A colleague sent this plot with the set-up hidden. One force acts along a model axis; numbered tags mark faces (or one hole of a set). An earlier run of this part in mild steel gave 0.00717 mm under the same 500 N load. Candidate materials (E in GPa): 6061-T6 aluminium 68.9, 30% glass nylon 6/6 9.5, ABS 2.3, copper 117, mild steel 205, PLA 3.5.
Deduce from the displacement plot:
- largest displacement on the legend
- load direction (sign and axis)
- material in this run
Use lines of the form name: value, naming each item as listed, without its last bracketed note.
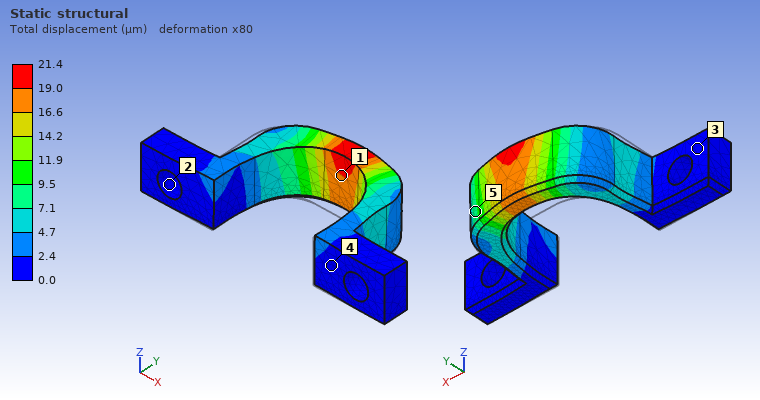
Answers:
largest displacement on the legend: 21.4 µm
load direction: +Y
material in this run: 6061-T6 aluminium
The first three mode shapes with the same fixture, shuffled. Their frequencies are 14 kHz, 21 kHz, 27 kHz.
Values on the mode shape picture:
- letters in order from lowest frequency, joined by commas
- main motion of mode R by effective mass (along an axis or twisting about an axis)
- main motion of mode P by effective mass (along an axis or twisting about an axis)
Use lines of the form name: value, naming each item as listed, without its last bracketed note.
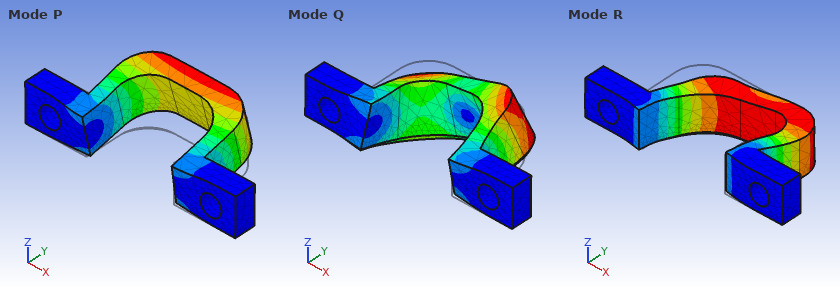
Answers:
letters in order from lowest frequency, joined by commas: P, R, Q
main motion of mode R by effective mass: along X
main motion of mode P by effective mass: along Z
